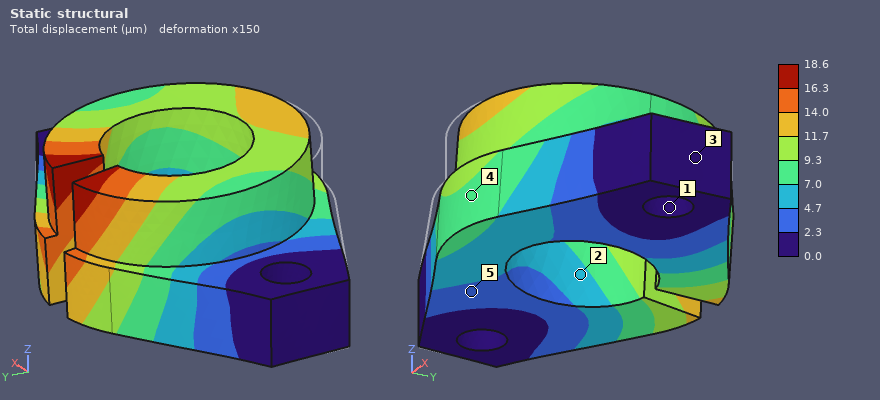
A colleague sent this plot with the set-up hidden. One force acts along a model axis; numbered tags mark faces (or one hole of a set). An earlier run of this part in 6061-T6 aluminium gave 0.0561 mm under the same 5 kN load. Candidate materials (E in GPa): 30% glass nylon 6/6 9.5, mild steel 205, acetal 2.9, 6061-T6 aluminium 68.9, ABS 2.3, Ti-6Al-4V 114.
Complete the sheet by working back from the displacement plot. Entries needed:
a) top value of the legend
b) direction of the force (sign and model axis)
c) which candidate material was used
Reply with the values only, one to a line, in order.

18.6 µm
+Y
mild steel
